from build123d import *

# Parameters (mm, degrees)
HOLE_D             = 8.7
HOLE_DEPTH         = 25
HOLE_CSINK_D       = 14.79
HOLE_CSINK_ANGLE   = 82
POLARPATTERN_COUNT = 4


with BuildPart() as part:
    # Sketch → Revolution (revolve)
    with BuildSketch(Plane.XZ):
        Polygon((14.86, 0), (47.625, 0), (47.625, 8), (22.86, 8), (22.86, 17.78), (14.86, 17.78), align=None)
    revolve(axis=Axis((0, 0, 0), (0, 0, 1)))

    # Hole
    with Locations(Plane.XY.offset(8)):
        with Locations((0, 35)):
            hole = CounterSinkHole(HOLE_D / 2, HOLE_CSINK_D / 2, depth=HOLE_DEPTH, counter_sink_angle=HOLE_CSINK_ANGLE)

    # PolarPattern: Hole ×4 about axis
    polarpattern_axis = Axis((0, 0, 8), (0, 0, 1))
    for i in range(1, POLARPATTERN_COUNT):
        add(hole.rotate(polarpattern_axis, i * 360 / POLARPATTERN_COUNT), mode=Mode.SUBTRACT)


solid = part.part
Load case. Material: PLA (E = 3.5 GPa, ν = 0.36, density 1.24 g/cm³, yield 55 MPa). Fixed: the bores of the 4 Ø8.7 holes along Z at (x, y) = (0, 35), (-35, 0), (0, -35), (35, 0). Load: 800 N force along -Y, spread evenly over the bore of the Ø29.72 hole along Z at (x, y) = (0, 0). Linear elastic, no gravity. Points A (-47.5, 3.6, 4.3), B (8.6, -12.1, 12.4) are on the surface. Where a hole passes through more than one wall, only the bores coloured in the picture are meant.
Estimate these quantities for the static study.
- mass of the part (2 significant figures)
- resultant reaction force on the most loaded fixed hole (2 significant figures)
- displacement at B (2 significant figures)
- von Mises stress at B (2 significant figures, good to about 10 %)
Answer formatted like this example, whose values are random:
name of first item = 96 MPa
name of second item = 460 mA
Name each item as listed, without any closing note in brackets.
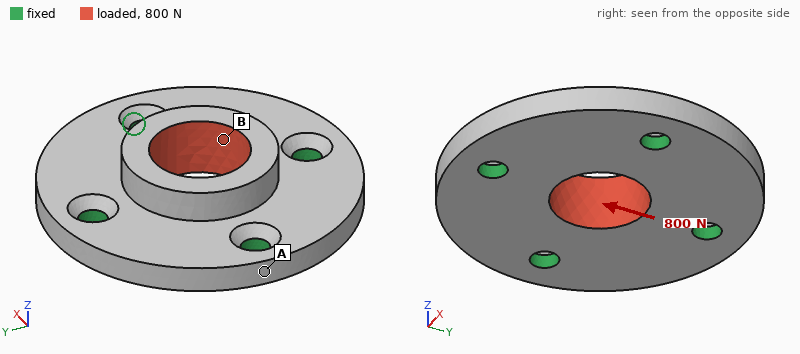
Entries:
mass of the part = 72 g
resultant reaction force on the most loaded fixed hole = 260 N
displacement at B = 13 µm
von Mises stress at B = 0.99 MPa
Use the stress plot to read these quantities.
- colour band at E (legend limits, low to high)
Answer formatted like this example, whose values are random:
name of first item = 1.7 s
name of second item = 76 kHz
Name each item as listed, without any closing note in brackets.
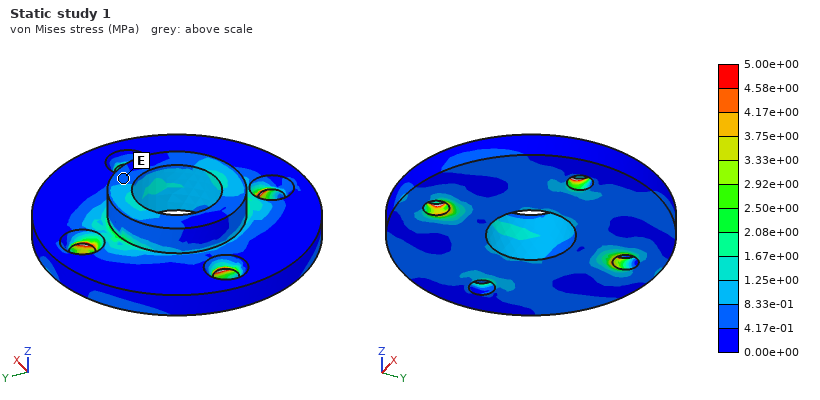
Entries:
colour band at E = 4.17e-01 to 8.33e-01 MPa
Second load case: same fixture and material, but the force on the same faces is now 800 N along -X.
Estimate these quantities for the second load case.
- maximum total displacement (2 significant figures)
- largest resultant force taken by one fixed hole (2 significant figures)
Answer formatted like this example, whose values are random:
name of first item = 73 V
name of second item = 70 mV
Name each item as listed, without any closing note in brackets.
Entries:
maximum total displacement = 16 µm
largest resultant force taken by one fixed hole = 260 N
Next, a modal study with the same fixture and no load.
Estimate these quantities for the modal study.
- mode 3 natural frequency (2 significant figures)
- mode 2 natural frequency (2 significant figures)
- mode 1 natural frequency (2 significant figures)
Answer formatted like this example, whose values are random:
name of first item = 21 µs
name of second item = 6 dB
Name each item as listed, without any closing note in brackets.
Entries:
mode 3 natural frequency = 3300 Hz
mode 2 natural frequency = 3300 Hz
mode 1 natural frequency = 3000 Hz
